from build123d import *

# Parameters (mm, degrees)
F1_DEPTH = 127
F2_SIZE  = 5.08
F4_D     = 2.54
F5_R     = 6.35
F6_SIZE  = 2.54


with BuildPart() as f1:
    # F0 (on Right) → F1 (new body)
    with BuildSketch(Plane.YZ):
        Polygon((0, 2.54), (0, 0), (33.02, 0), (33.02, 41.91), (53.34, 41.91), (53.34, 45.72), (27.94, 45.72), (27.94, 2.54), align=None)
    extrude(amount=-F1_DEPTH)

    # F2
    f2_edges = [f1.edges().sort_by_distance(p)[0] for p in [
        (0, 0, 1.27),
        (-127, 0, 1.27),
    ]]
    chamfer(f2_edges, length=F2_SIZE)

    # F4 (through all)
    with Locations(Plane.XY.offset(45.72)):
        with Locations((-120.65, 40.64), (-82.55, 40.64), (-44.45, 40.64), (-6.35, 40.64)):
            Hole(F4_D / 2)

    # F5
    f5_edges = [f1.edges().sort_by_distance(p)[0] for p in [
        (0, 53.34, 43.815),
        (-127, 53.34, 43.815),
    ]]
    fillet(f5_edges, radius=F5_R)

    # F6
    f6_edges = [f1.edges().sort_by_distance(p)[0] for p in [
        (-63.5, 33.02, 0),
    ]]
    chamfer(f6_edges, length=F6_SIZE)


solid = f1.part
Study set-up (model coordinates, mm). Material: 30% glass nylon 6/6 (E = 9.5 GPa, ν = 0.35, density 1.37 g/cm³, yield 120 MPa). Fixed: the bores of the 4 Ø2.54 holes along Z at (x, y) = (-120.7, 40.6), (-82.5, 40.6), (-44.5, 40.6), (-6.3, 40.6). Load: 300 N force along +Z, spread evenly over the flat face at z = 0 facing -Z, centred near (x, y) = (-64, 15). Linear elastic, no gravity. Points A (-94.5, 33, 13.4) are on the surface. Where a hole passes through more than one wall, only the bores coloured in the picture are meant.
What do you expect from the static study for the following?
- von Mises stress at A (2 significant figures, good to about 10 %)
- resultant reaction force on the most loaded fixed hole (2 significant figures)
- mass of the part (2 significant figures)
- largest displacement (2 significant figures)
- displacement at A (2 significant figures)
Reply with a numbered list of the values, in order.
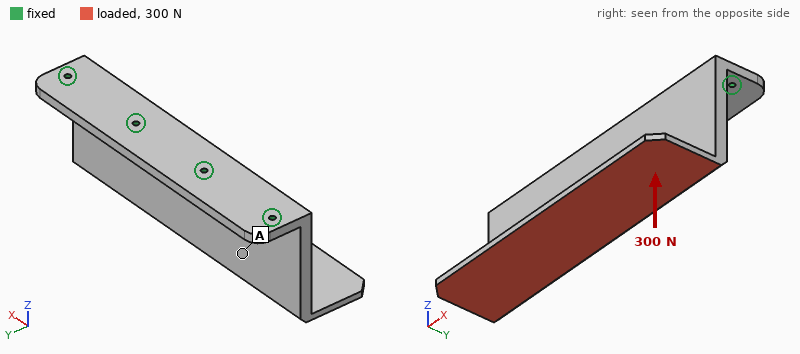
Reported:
1. 7.1 MPa
2. 95 N
3. 65 g
4. 1.7 mm
5. 0.60 mm
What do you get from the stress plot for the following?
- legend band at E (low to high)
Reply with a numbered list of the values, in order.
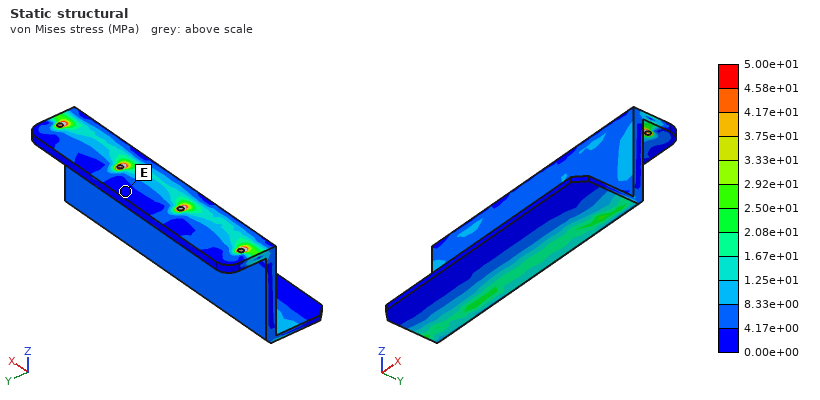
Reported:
1. 0.00e+00 to 4.17e+00 MPa
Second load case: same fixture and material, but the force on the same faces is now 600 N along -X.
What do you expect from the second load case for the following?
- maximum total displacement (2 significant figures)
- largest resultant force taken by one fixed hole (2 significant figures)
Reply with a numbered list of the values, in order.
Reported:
1. 0.63 mm
2. 260 N
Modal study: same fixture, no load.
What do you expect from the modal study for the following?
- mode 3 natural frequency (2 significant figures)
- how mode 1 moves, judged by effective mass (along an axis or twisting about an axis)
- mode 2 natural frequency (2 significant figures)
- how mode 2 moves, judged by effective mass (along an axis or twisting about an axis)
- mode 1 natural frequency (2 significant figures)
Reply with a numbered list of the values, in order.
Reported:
1. 1300 Hz
2. along Y
3. 680 Hz
4. twisting about Z
5. 380 Hz
